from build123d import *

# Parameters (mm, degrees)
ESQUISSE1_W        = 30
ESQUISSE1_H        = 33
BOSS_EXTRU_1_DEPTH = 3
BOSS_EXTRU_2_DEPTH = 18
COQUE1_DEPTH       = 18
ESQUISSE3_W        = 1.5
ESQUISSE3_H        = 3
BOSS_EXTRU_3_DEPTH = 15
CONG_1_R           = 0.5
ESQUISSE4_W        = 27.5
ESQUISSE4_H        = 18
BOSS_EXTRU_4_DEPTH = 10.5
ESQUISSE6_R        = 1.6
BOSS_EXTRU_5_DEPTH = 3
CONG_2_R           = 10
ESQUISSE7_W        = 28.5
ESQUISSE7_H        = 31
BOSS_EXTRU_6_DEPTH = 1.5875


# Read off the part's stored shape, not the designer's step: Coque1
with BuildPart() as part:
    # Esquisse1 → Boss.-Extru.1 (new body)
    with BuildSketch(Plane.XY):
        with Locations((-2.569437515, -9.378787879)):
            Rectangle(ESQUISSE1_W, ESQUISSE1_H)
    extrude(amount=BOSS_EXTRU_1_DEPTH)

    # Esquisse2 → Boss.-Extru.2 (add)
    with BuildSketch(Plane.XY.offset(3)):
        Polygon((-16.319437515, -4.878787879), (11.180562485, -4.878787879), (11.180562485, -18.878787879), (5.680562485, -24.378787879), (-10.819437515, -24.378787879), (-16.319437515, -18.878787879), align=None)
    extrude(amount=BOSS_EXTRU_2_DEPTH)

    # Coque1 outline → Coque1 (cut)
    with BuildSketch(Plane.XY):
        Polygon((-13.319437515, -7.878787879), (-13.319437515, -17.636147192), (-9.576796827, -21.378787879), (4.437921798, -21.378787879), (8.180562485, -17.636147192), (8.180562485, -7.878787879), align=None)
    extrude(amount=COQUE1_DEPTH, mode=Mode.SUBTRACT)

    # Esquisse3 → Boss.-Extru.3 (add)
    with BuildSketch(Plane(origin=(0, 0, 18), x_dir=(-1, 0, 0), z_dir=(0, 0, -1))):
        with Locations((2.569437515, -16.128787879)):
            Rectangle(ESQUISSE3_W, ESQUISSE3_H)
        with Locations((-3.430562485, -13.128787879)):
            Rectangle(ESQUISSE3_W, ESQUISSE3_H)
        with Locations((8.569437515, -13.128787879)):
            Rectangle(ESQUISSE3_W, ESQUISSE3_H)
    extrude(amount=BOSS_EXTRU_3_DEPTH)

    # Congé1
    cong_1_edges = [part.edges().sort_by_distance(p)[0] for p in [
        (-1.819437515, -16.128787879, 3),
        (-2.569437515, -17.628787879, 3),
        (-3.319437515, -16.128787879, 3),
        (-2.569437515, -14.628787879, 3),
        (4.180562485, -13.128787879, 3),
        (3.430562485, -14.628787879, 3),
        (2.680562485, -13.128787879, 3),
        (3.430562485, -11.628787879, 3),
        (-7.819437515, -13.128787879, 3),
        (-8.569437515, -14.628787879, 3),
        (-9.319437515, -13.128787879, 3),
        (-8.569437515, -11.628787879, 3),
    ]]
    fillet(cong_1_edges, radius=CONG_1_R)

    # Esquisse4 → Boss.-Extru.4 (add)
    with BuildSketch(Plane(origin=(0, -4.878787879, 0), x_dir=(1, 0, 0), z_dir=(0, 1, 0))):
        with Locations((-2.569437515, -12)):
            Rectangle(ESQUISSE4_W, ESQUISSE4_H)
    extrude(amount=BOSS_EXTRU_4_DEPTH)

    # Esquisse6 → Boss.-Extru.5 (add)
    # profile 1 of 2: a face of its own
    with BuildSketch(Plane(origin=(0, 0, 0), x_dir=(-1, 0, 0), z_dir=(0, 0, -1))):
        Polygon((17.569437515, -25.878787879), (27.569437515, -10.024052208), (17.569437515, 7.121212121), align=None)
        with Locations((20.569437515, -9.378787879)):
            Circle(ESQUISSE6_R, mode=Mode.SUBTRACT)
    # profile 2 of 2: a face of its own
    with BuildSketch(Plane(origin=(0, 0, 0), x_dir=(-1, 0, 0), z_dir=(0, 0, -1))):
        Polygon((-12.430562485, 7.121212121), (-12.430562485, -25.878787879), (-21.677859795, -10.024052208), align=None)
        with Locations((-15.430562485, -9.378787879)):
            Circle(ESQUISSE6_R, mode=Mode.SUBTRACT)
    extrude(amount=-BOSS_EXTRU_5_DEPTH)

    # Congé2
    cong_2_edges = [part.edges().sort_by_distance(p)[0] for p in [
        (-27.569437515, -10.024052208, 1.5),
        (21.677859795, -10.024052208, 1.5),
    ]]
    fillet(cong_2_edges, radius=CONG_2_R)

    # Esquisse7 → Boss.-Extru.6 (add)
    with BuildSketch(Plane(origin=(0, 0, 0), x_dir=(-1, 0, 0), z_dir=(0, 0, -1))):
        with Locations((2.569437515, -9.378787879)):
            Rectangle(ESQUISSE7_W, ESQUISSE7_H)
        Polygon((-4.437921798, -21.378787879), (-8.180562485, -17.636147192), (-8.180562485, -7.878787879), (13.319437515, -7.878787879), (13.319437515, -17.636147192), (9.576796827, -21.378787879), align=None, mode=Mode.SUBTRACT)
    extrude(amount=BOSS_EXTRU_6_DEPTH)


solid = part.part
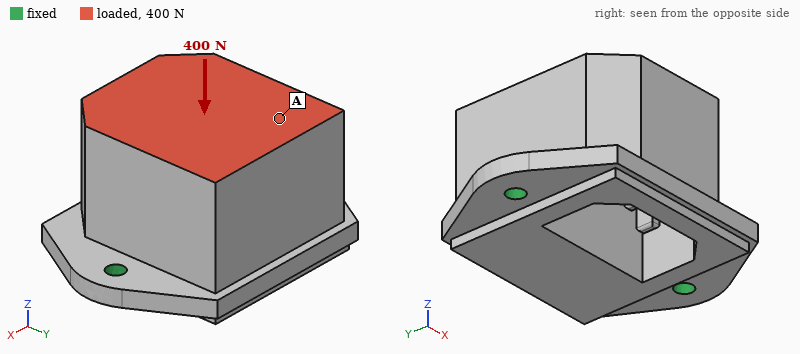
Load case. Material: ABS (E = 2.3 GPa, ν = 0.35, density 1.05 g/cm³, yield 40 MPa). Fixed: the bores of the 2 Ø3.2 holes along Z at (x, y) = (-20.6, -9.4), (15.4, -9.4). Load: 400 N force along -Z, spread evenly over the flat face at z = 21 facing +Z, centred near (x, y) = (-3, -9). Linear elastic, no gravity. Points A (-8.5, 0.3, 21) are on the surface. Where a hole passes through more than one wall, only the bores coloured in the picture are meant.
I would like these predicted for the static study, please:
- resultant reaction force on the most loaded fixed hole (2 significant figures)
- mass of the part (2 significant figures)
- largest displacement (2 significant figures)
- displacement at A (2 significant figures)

210 N
15 g
0.12 mm
0.11 mm
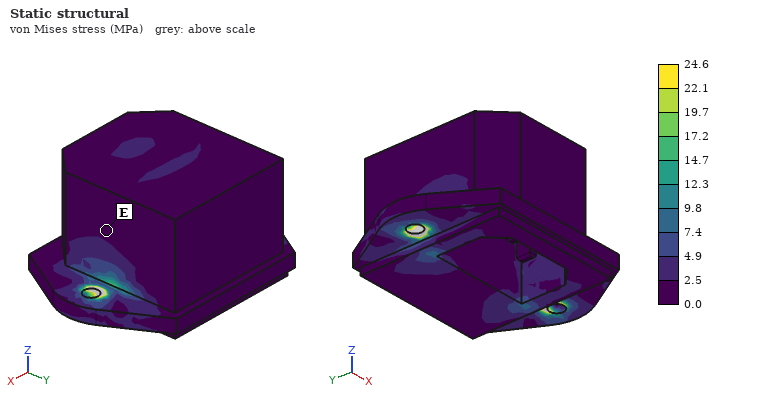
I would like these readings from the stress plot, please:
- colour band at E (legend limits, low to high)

0.0 to 2.5 MPa
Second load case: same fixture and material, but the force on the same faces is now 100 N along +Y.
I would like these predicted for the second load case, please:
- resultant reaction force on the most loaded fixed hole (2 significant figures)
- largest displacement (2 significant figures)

51 N
0.70 mm
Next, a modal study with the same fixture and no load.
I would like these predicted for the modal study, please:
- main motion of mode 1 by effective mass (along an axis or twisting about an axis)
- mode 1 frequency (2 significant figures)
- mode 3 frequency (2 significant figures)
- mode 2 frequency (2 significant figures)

along Y
770 Hz
1600 Hz
1600 Hz
